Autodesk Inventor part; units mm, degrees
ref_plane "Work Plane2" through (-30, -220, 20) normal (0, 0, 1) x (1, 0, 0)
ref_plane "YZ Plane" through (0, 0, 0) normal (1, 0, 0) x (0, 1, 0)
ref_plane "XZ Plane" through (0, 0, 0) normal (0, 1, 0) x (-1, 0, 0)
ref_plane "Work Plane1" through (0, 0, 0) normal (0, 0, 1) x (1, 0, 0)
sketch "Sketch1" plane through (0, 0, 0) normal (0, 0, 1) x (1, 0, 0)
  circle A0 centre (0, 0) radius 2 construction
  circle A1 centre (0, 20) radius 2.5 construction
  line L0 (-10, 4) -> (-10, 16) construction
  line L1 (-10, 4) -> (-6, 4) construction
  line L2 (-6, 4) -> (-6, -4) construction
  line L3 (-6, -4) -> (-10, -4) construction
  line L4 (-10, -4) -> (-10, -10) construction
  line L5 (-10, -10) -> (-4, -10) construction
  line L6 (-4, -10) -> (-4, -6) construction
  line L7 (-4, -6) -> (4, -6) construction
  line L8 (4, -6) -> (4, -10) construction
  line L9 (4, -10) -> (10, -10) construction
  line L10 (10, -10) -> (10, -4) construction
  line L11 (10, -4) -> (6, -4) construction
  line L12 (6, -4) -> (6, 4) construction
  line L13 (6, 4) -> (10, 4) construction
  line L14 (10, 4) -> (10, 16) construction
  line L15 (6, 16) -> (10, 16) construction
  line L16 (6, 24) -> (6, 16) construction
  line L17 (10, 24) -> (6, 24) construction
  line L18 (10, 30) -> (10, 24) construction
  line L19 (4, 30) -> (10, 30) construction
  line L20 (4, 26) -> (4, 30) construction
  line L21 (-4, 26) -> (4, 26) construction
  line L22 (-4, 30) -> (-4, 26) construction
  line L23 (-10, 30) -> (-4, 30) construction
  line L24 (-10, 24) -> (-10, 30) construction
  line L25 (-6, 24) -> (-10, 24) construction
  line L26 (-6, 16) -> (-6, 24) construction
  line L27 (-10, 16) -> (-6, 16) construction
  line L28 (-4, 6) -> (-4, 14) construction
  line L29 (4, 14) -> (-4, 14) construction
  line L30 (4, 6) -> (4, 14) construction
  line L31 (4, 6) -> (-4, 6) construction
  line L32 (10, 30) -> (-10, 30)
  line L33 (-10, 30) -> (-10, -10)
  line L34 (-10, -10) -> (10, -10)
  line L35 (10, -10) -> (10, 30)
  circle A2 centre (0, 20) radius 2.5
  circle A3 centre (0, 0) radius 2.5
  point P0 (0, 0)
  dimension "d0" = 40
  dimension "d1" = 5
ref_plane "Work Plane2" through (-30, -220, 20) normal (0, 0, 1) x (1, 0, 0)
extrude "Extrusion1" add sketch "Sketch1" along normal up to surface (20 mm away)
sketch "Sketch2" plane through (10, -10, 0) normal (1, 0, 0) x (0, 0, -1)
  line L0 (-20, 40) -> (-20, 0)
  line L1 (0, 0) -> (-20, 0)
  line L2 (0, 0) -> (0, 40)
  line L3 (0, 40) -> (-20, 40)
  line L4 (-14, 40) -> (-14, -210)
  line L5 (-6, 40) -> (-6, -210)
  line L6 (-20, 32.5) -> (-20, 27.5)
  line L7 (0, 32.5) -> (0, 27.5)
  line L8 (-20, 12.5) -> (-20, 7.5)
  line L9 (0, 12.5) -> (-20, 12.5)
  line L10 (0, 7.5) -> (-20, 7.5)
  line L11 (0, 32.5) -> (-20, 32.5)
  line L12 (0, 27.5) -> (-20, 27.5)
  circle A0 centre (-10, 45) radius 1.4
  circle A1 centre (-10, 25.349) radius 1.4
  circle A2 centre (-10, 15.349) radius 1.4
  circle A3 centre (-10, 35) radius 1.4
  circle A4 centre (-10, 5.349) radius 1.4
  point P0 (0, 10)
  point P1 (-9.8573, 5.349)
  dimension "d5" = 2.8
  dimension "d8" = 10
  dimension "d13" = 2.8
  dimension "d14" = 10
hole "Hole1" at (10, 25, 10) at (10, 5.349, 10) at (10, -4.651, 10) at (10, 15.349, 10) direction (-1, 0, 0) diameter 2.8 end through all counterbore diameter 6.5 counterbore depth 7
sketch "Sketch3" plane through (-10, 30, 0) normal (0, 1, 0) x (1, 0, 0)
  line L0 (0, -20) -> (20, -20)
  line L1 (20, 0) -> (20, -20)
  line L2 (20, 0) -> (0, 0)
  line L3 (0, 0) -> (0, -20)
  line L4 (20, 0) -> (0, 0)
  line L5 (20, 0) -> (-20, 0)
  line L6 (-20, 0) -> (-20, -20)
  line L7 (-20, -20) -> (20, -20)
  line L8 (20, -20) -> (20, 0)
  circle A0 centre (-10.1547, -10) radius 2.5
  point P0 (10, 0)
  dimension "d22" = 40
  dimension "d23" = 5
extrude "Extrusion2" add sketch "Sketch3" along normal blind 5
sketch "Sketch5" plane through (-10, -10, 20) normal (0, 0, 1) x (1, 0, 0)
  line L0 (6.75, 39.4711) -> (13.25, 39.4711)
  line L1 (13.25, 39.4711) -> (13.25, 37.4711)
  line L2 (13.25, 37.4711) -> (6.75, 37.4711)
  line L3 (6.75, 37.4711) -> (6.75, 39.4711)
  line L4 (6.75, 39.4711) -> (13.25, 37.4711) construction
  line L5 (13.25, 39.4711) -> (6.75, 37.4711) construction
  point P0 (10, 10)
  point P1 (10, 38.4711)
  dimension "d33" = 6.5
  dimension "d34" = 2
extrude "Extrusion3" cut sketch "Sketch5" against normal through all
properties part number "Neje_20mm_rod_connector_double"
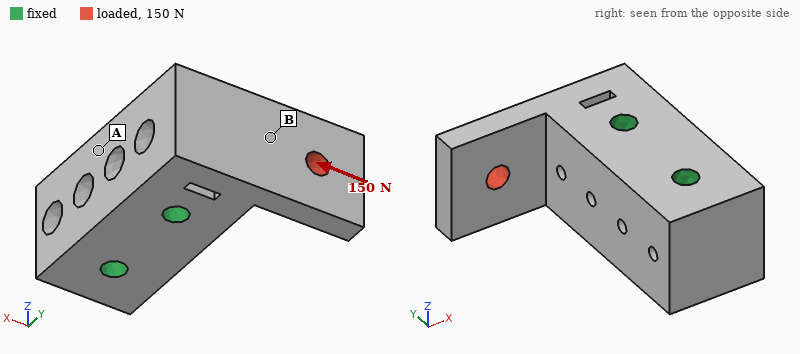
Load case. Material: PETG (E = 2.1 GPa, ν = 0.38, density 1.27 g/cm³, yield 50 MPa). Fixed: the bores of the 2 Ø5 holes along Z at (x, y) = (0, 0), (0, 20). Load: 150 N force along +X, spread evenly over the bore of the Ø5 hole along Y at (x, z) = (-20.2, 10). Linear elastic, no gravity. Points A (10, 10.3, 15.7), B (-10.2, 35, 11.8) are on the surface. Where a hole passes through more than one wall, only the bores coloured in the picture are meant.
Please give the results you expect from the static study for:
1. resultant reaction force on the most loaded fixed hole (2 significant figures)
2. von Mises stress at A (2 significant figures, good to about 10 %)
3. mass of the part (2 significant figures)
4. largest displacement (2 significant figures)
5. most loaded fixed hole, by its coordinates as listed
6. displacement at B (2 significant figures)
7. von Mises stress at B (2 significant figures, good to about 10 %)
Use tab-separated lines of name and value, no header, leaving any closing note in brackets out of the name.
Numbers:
resultant reaction force on the most loaded fixed hole	200 N
von Mises stress at A	0.56 MPa
mass of the part	22 g
largest displacement	77 µm
most loaded fixed hole, by its coordinates as listed	(0, 20)
displacement at B	35 µm
von Mises stress at B	1.9 MPa
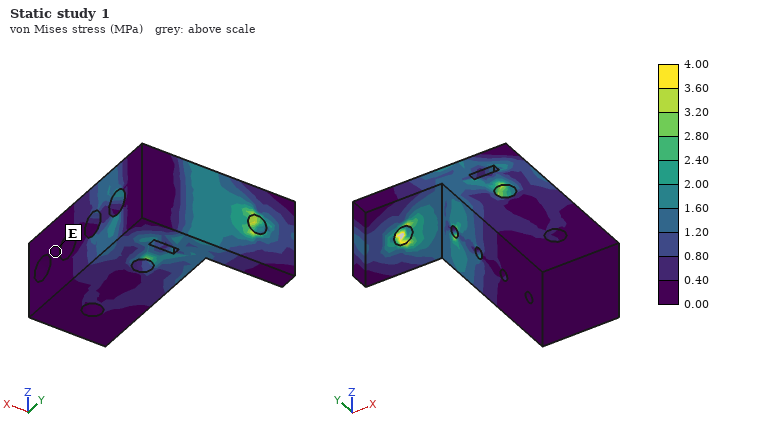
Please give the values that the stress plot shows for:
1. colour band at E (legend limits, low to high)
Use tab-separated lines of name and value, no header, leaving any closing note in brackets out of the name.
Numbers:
colour band at E	0.00 to 0.40 MPa
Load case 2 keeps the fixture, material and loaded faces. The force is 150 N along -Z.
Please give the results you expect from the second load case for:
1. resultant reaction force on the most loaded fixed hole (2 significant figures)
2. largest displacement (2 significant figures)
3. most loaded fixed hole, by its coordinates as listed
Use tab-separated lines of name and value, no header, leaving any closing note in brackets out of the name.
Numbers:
resultant reaction force on the most loaded fixed hole	150 N
largest displacement	0.18 mm
most loaded fixed hole, by its coordinates as listed	(0, 20)
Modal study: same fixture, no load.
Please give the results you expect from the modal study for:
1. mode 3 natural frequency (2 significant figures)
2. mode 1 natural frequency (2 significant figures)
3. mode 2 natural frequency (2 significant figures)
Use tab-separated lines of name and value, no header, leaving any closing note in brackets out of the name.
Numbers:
mode 3 natural frequency	4400 Hz
mode 1 natural frequency	1900 Hz
mode 2 natural frequency	3300 Hz
